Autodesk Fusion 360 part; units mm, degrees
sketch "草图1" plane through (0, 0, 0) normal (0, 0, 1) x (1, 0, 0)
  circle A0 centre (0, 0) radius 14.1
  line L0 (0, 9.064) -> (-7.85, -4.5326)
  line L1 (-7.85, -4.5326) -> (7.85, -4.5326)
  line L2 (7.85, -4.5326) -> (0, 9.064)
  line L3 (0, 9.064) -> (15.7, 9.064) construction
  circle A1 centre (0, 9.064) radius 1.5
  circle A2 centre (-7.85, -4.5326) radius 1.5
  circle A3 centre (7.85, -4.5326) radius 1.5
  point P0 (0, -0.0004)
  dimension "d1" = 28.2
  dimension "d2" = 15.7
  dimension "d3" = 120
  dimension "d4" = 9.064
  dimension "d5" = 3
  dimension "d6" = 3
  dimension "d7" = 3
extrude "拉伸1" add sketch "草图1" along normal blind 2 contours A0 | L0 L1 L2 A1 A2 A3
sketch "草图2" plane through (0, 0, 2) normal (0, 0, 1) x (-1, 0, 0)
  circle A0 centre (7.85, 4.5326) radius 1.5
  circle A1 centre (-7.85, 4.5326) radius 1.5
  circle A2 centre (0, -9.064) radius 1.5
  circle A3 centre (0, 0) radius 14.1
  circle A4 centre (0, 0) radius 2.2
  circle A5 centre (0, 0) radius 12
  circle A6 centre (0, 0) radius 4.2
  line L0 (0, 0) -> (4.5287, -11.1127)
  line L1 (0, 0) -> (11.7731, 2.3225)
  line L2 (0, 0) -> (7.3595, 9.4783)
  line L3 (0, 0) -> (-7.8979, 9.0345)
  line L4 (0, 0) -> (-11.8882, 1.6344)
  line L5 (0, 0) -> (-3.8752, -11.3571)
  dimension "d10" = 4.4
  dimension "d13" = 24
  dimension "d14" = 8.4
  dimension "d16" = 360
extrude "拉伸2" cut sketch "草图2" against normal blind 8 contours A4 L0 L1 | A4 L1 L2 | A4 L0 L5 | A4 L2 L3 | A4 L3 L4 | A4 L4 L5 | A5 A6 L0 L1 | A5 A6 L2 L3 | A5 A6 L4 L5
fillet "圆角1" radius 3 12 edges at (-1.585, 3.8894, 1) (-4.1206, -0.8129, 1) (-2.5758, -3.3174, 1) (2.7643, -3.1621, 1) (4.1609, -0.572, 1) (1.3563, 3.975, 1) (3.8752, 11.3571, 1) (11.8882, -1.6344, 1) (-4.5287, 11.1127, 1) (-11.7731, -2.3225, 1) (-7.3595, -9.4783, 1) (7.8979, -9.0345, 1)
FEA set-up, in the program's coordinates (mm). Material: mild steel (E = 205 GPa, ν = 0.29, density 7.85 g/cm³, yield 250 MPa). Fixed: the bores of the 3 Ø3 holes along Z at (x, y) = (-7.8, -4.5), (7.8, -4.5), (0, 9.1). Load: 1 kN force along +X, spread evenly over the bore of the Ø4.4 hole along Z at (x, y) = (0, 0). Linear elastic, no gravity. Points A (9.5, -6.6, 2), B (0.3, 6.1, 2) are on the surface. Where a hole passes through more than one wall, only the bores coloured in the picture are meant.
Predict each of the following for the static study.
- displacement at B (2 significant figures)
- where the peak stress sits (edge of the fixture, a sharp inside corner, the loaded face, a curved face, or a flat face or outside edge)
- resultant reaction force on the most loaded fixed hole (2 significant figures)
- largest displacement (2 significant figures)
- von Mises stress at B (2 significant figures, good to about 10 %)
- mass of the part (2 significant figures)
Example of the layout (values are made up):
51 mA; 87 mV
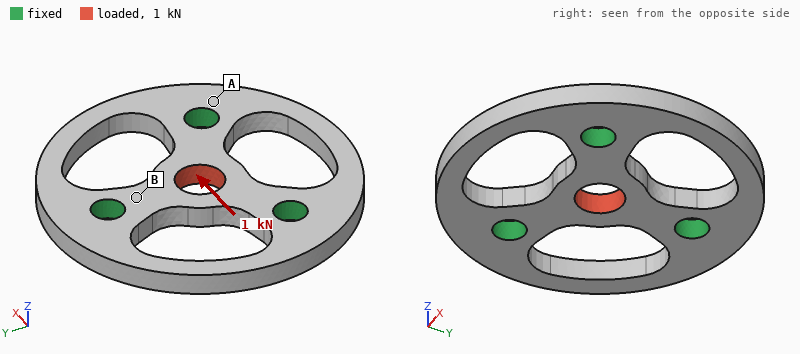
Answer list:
0.94 µm; the loaded face; 420 N; 4.5 µm; 43 MPa; 5.5 g
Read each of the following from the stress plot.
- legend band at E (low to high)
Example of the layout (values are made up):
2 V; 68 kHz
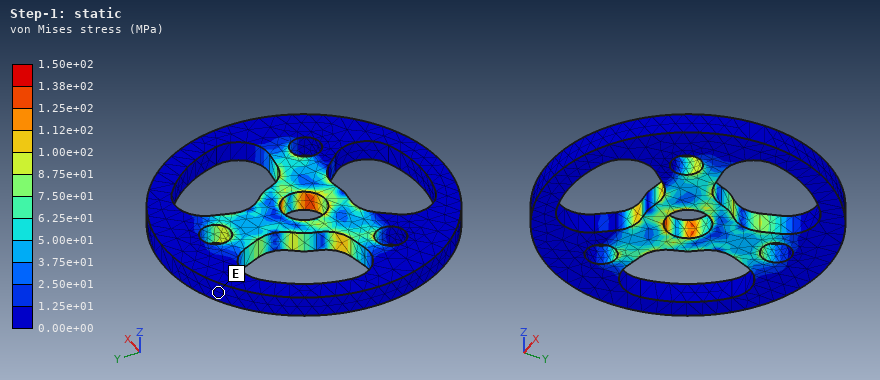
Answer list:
0.00e+00 to 1.25e+01 MPa
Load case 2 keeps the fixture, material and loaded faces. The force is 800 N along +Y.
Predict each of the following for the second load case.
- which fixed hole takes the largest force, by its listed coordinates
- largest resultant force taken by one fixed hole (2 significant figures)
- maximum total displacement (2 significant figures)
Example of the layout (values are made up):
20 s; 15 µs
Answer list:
(0, 9.1); 380 N; 3.9 µm
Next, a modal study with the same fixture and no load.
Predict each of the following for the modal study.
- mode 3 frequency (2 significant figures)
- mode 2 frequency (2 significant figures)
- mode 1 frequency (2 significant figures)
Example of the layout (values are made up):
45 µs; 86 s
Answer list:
19 kHz; 19 kHz; 19 kHz
